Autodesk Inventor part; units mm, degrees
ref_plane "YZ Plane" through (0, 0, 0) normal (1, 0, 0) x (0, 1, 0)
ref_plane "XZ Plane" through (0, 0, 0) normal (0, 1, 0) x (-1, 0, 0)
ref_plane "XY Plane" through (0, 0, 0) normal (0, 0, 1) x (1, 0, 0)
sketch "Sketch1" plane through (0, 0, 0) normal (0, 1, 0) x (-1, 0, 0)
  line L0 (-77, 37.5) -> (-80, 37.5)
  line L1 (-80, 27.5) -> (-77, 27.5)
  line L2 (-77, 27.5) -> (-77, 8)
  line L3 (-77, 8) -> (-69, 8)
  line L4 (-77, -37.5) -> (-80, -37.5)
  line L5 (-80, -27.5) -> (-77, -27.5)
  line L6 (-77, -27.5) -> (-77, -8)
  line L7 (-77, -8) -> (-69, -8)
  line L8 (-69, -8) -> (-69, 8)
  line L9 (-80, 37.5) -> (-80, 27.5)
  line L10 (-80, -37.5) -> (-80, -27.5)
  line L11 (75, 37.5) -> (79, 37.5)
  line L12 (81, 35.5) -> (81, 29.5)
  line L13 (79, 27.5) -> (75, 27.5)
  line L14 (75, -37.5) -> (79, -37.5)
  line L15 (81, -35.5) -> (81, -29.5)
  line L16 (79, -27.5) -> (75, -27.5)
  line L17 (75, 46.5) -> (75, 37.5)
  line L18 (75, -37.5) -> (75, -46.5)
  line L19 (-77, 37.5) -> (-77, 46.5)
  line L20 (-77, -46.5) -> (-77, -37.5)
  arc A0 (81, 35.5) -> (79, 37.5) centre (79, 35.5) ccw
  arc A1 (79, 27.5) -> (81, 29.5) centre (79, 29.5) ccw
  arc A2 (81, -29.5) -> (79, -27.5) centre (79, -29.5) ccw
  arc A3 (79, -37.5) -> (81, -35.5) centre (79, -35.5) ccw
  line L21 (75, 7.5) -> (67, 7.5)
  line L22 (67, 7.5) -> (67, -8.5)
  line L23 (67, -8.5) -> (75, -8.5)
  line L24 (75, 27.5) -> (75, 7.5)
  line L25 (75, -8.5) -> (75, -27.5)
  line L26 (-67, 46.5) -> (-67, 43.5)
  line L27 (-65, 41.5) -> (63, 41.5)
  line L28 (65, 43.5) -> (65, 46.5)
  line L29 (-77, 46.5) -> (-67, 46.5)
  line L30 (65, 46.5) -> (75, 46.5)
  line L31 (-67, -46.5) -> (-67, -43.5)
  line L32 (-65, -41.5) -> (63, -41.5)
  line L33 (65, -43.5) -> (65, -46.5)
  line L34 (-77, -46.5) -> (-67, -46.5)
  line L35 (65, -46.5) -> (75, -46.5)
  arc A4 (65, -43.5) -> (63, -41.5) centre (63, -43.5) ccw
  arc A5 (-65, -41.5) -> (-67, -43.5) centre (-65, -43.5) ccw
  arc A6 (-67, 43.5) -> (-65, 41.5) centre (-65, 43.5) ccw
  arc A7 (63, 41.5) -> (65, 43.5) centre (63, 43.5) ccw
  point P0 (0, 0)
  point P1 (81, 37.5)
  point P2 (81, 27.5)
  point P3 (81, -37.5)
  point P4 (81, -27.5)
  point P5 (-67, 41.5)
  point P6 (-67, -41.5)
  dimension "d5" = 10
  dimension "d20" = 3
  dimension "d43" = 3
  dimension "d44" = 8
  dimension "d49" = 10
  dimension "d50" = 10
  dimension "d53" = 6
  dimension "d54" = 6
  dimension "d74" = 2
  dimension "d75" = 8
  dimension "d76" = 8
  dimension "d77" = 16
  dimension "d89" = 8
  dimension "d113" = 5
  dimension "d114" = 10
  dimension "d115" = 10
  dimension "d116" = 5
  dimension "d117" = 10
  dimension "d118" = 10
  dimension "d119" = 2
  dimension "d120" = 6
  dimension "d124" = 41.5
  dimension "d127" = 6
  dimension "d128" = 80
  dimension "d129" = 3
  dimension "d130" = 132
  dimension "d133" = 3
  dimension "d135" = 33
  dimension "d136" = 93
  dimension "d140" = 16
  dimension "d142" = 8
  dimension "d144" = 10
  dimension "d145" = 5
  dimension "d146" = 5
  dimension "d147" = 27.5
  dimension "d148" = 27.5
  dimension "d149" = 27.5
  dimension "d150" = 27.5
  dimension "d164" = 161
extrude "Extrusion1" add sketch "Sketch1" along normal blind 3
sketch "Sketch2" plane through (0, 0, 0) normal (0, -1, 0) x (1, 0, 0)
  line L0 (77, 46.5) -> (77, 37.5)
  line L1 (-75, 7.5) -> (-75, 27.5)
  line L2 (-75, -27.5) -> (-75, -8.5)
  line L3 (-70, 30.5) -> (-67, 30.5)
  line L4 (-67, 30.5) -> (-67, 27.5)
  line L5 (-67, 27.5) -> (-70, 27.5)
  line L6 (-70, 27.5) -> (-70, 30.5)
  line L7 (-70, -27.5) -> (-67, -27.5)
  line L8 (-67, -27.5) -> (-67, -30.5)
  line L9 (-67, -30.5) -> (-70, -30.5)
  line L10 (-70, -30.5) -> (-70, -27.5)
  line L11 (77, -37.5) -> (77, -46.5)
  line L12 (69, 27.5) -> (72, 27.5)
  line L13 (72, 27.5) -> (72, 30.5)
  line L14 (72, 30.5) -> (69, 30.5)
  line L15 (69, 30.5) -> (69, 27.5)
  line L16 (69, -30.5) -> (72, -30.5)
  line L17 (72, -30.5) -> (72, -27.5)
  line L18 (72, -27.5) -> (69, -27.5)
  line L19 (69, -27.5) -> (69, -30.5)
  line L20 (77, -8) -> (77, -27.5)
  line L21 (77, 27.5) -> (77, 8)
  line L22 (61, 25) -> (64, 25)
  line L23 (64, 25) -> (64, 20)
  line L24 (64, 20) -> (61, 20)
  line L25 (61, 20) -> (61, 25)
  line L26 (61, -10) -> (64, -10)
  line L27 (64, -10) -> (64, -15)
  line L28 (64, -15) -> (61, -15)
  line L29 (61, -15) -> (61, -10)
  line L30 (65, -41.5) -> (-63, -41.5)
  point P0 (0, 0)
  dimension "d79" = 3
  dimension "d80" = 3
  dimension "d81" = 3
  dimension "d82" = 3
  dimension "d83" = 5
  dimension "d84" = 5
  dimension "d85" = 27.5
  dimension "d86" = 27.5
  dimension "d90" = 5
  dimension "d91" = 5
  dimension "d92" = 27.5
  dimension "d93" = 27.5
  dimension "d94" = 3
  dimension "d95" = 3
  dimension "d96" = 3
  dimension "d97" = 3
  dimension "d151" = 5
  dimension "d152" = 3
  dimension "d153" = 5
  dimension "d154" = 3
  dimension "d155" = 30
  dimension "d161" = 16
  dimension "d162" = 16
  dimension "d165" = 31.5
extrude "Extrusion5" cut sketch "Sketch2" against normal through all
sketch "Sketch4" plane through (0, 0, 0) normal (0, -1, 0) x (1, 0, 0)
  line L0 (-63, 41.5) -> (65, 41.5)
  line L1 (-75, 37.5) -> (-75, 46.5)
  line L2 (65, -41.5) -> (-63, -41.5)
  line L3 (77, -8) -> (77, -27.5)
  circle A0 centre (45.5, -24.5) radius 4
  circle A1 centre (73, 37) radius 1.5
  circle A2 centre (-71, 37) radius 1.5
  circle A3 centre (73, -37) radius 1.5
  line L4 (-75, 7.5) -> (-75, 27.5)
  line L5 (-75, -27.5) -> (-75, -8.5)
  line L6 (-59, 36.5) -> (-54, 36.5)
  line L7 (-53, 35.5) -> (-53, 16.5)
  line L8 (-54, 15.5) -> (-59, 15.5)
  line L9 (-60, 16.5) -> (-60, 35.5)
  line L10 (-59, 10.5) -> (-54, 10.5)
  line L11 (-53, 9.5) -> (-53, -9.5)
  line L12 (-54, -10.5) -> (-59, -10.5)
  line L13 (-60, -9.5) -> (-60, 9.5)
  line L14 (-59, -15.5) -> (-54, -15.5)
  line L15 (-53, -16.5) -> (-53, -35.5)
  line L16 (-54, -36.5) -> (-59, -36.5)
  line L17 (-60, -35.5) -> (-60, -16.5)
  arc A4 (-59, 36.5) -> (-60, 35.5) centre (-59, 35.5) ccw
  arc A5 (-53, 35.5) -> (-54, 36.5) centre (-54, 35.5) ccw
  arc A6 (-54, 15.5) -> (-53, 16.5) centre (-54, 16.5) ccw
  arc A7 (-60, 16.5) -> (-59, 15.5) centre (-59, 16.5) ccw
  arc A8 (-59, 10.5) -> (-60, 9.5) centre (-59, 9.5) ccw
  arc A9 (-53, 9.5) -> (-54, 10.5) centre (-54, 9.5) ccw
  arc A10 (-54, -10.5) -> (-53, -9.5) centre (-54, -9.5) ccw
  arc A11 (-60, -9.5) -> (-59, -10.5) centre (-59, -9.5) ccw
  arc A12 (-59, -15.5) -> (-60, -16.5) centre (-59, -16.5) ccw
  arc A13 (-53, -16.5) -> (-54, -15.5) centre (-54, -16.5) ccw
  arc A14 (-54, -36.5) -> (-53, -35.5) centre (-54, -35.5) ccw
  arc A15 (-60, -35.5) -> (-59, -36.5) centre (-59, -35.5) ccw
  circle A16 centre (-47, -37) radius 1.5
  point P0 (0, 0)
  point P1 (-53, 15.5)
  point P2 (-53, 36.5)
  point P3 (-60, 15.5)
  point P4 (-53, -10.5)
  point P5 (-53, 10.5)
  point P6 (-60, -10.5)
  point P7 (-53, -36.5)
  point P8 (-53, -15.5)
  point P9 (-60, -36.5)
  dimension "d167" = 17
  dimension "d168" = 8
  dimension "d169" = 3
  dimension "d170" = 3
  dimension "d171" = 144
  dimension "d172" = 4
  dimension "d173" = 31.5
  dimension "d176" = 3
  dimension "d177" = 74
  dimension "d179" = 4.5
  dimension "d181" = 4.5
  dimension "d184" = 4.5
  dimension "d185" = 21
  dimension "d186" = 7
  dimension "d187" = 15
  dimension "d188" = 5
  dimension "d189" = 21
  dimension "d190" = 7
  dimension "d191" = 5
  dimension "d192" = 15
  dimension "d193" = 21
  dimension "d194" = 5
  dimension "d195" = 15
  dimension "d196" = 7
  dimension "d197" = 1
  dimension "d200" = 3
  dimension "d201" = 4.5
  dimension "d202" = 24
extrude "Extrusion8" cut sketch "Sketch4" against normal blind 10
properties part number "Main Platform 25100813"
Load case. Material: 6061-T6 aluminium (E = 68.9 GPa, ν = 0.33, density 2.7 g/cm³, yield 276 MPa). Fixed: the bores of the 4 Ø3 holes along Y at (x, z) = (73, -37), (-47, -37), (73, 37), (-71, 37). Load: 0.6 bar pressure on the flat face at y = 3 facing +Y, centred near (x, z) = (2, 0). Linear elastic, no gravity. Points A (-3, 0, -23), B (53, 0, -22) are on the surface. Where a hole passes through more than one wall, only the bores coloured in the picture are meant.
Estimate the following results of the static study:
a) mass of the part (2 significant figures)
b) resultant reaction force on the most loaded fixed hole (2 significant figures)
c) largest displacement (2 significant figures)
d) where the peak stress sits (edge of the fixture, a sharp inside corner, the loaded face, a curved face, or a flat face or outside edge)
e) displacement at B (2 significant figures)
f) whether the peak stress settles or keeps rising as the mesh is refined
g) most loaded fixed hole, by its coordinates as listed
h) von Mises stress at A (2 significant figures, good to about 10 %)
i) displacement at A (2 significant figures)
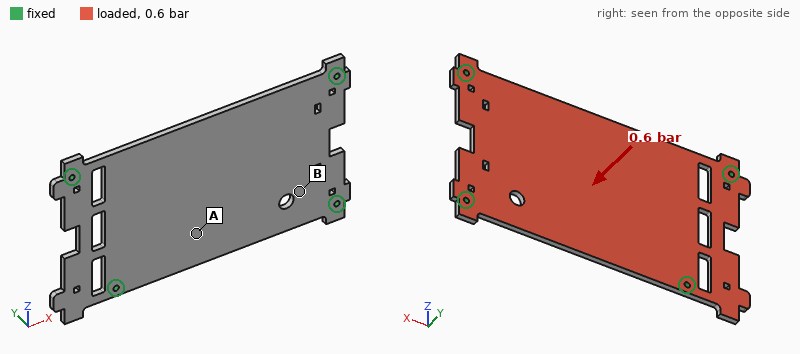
98 g
240 N
0.62 mm
edge of the fixture
0.17 mm
keeps rising
(-47, -37)
29 MPa
0.36 mm
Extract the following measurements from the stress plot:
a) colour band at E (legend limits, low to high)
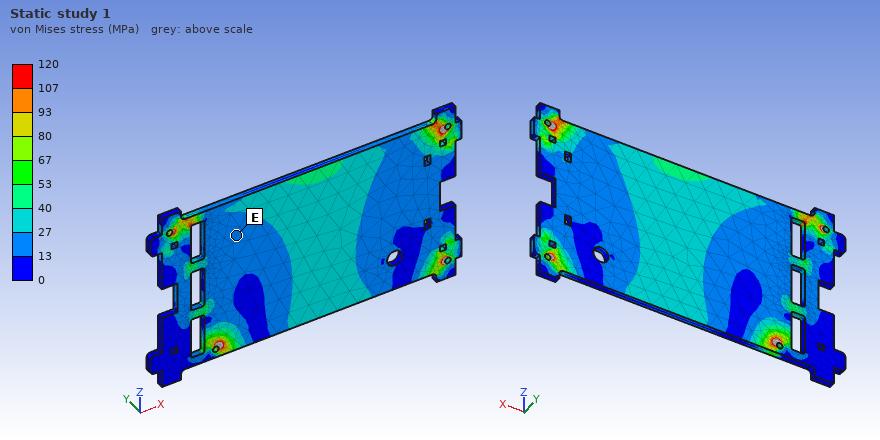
13 to 27 MPa
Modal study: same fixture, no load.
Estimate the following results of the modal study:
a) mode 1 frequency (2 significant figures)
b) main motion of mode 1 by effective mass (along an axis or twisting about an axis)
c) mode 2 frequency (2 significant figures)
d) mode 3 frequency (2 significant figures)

690 Hz
along Y
1300 Hz
1700 Hz
